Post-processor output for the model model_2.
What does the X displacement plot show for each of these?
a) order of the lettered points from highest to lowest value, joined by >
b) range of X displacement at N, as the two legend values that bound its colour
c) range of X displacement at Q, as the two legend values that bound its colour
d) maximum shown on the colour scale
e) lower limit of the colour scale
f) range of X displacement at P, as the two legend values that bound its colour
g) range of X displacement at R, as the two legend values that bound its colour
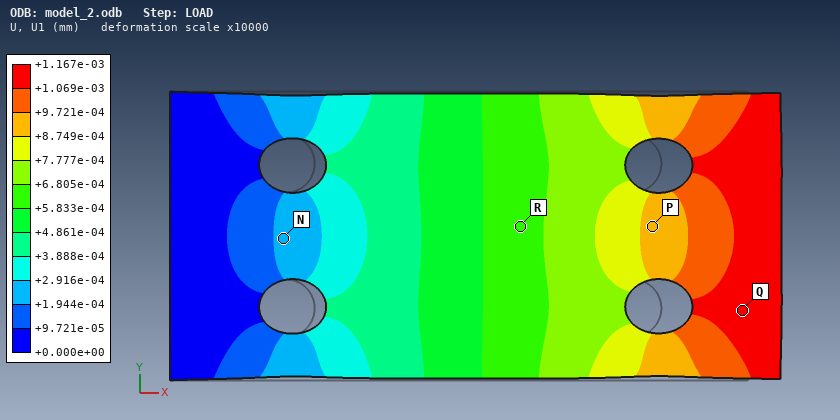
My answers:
Q > P > R > N
+1.944e-04 to +2.916e-04 mm
+1.069e-03 to +1.167e-03 mm
+1.167e-03 mm
+0.000e+00 mm
+8.749e-04 to +9.721e-04 mm
+5.833e-04 to +6.805e-04 mm
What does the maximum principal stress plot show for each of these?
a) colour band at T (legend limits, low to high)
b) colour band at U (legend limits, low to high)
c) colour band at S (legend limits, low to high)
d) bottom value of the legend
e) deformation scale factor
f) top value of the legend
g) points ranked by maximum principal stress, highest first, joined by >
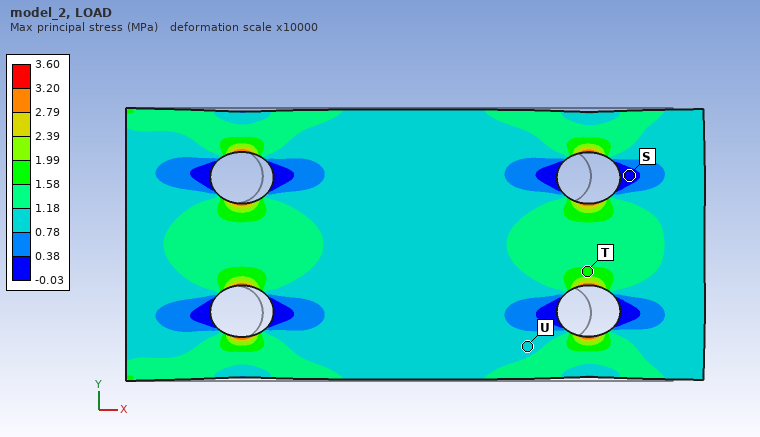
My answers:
1.58 to 1.99 MPa
0.78 to 1.18 MPa
-0.03 to 0.38 MPa
-0.03 MPa
10000
3.60 MPa
T > U > S
